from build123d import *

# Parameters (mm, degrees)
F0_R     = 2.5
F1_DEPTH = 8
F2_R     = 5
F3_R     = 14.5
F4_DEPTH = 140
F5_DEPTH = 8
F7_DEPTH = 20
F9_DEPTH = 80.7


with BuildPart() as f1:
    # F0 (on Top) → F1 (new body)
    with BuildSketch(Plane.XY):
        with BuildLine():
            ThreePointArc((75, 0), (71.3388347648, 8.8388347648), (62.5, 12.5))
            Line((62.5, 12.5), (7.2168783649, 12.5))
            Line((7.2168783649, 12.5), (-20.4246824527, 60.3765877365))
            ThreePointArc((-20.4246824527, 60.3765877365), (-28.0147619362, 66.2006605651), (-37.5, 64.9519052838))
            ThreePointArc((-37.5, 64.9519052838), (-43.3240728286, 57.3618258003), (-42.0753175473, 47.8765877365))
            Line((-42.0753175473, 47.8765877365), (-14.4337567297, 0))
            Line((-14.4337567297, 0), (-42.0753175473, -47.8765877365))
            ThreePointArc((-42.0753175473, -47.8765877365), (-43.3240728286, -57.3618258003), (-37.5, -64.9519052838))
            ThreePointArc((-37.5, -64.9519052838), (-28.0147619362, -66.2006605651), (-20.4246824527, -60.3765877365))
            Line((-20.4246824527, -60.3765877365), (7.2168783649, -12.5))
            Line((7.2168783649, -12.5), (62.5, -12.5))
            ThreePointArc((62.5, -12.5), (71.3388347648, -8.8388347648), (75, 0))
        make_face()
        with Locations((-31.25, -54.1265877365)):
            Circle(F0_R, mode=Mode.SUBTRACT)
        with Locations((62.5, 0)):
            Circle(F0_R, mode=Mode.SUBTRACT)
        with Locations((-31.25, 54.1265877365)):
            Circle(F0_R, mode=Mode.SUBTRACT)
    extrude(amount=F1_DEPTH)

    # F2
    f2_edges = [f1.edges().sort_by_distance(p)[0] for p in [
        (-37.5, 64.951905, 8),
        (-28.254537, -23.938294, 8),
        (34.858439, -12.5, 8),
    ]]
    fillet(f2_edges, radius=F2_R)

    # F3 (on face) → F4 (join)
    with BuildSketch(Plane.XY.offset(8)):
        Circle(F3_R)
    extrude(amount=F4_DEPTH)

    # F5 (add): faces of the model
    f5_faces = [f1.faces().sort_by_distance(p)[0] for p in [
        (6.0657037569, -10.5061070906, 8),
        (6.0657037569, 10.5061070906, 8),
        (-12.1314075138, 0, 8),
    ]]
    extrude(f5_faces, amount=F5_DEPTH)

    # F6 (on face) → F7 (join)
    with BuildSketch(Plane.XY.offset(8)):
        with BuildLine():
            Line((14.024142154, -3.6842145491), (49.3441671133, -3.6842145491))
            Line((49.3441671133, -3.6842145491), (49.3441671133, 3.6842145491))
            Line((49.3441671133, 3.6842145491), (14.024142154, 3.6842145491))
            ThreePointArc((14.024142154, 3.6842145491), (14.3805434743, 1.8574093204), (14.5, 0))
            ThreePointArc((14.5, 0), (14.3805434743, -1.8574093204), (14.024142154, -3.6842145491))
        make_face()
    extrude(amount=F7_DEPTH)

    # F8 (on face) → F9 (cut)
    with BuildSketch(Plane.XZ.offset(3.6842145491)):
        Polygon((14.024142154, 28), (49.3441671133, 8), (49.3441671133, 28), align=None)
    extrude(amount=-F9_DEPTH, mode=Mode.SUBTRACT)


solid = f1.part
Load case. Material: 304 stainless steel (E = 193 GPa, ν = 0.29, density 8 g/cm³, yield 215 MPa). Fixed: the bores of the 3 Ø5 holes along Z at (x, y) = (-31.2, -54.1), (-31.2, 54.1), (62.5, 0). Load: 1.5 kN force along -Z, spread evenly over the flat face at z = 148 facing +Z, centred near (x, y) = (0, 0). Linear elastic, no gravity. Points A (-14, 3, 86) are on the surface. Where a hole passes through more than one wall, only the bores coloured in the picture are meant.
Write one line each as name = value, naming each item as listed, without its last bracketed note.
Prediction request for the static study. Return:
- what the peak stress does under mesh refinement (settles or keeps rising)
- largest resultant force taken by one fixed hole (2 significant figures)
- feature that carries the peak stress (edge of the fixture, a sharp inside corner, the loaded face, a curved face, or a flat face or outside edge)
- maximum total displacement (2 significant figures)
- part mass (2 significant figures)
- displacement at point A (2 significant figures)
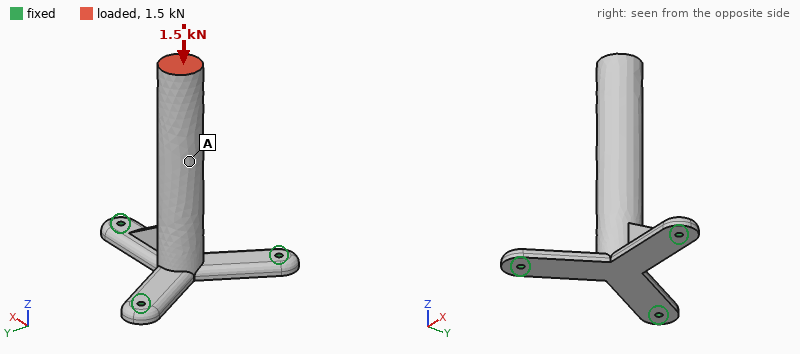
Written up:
what the peak stress does under mesh refinement = keeps rising
largest resultant force taken by one fixed hole = 550 N
feature that carries the peak stress = edge of the fixture
maximum total displacement = 67 µm
part mass = 1.1 kg
displacement at point A = 48 µm
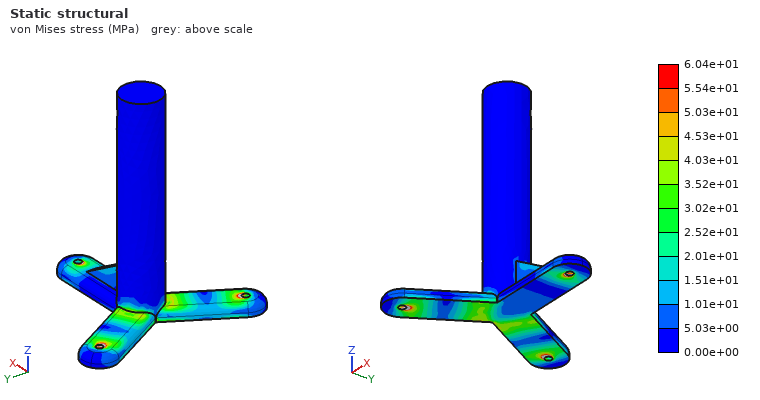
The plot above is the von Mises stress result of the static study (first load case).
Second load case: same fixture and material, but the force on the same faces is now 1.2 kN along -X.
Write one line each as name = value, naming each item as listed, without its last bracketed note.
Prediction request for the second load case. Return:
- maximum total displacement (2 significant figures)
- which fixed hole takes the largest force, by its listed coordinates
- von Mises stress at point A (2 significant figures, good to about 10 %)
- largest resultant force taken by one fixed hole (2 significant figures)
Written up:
maximum total displacement = 0.40 mm
which fixed hole takes the largest force, by its listed coordinates = (62.5, 0)
von Mises stress at point A = 30 MPa
largest resultant force taken by one fixed hole = 2.7 kN
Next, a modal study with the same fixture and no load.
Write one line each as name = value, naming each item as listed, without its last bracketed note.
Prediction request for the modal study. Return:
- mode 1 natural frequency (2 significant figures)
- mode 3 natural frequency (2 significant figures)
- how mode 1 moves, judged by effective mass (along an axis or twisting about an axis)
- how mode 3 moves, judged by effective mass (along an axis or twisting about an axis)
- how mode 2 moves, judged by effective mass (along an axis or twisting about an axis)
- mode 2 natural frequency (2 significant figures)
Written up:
mode 1 natural frequency = 410 Hz
mode 3 natural frequency = 1500 Hz
how mode 1 moves, judged by effective mass = along Y
how mode 3 moves, judged by effective mass = along Z
how mode 2 moves, judged by effective mass = along X
mode 2 natural frequency = 570 Hz
